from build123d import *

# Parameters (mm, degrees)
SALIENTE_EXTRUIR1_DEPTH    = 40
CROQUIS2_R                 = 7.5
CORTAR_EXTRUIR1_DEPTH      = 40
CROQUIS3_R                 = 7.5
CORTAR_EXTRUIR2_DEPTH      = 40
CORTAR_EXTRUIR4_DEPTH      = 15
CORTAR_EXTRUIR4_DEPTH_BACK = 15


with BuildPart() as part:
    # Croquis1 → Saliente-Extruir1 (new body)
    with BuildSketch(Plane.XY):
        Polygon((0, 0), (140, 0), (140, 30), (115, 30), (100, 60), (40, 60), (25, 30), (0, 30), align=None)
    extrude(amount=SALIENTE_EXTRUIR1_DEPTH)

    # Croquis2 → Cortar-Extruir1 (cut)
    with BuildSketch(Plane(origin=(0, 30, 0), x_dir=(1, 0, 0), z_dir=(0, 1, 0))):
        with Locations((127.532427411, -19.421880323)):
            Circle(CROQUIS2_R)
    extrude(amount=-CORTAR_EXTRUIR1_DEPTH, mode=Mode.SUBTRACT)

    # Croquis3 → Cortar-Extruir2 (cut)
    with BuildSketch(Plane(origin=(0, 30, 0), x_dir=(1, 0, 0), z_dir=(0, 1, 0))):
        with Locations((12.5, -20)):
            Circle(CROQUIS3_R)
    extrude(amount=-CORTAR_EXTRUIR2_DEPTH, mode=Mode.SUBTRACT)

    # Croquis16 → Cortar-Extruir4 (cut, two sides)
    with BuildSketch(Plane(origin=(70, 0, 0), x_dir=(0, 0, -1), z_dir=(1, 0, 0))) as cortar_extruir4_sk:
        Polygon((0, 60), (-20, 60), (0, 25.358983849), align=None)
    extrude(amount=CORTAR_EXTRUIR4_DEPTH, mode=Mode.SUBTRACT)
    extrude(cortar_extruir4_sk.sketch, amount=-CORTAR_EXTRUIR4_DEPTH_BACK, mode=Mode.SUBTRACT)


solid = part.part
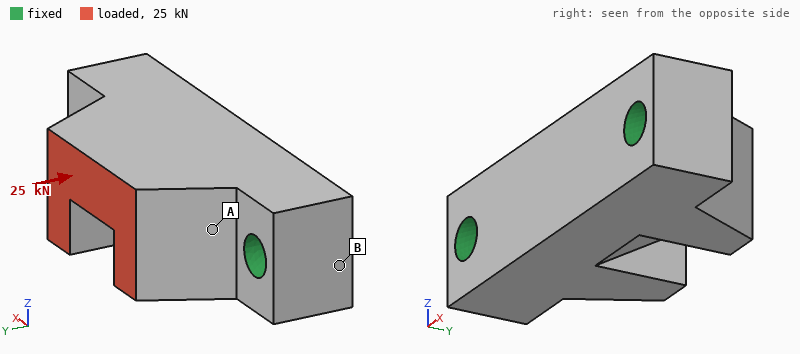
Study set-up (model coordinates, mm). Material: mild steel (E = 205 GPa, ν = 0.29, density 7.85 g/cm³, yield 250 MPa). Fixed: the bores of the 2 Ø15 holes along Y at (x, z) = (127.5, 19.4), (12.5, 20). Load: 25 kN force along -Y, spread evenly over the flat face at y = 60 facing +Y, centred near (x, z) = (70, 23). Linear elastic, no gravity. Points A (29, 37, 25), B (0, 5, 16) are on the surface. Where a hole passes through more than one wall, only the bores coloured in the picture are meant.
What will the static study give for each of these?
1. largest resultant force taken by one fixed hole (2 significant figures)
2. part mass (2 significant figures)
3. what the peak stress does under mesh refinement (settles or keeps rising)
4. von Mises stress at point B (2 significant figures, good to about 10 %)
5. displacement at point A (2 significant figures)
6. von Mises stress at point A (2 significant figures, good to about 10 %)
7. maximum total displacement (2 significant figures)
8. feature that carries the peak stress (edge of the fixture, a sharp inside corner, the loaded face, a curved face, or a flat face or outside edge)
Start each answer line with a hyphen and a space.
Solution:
- 14 kN
- 1.9 kg
- keeps rising
- 6.3 MPa
- 3.9 µm
- 22 MPa
- 11 µm
- edge of the fixture
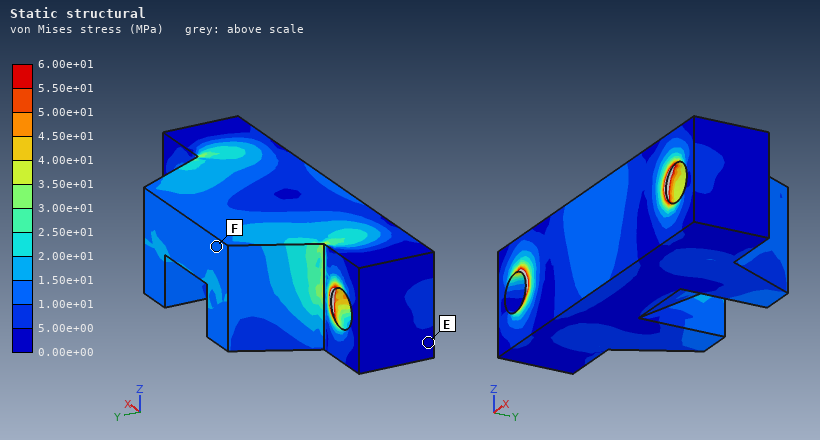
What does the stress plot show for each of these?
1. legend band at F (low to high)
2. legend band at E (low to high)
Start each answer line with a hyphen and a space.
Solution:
- 1.00e+01 to 1.50e+01 MPa
- 0.00e+00 to 5.00e+00 MPa
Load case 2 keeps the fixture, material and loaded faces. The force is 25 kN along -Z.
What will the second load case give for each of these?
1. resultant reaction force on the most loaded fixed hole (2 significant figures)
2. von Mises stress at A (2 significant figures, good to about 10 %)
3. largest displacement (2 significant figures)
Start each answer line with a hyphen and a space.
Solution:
- 13 kN
- 63 MPa
- 58 µm
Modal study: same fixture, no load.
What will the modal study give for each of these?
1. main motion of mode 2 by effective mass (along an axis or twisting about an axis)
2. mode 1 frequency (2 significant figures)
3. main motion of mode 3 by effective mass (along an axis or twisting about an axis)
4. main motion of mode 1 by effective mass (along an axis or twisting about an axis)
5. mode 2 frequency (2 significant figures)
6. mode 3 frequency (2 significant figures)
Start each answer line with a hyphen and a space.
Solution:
- along Y
- 5800 Hz
- along Z
- along Z
- 9200 Hz
- 10000 Hz
